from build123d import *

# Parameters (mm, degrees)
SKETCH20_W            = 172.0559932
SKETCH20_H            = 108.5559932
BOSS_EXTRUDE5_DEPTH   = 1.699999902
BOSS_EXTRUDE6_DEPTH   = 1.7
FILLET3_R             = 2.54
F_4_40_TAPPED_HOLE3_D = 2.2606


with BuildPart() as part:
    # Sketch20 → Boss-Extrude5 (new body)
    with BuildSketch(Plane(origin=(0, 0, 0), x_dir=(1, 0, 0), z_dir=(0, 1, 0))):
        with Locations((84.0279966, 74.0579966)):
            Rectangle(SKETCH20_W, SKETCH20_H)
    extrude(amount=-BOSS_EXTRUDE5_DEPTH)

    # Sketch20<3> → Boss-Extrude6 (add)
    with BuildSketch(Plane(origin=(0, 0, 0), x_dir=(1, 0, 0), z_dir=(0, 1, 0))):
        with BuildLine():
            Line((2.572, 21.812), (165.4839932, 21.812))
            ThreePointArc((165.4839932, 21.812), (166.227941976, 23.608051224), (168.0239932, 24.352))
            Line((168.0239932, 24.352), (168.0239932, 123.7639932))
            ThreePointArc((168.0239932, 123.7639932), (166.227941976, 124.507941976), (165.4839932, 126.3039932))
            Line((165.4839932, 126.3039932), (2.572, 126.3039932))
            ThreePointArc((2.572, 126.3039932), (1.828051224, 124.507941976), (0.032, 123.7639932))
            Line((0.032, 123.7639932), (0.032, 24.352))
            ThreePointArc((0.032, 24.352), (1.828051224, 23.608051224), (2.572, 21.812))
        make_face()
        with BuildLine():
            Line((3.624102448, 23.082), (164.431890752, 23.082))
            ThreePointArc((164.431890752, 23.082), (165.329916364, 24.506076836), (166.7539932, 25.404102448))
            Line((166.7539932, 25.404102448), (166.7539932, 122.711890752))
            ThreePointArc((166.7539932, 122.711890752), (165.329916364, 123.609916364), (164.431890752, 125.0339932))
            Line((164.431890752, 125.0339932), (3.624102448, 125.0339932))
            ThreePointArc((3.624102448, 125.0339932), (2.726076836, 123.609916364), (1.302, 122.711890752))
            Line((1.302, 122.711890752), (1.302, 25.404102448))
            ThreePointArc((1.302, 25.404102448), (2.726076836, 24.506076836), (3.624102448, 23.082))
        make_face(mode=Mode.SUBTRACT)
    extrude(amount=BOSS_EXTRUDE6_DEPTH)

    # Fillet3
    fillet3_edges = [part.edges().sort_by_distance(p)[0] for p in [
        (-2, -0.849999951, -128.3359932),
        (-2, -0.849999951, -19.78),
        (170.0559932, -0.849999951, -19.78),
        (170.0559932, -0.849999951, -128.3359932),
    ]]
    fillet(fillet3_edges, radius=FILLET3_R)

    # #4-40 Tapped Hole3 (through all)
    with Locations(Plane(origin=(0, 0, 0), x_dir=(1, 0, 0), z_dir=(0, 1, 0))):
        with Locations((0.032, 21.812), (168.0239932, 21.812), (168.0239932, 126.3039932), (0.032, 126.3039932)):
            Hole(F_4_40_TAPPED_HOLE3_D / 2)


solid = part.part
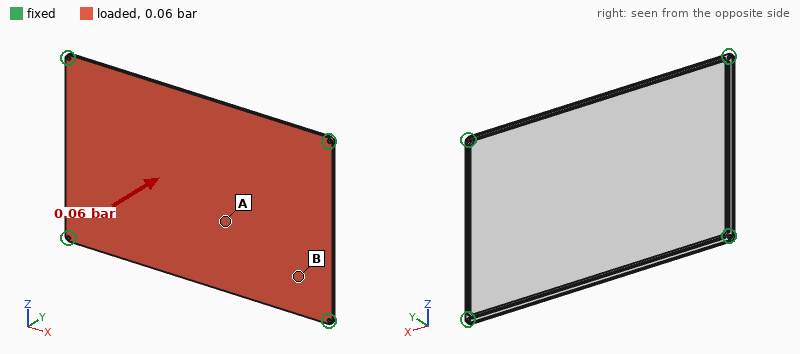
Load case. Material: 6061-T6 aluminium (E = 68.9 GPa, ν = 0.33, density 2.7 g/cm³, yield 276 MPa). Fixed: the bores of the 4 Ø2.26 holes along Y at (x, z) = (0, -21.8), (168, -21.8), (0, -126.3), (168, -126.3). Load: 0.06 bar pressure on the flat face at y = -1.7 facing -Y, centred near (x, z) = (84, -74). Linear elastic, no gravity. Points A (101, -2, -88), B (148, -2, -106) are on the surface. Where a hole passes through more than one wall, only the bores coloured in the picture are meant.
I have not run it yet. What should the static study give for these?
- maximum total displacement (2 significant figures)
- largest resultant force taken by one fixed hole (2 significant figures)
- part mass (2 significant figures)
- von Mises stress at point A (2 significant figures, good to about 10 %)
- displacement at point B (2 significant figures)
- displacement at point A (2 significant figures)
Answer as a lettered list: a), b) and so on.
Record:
a) 0.72 mm
b) 34 N
c) 89 g
d) 15 MPa
e) 0.24 mm
f) 0.68 mm
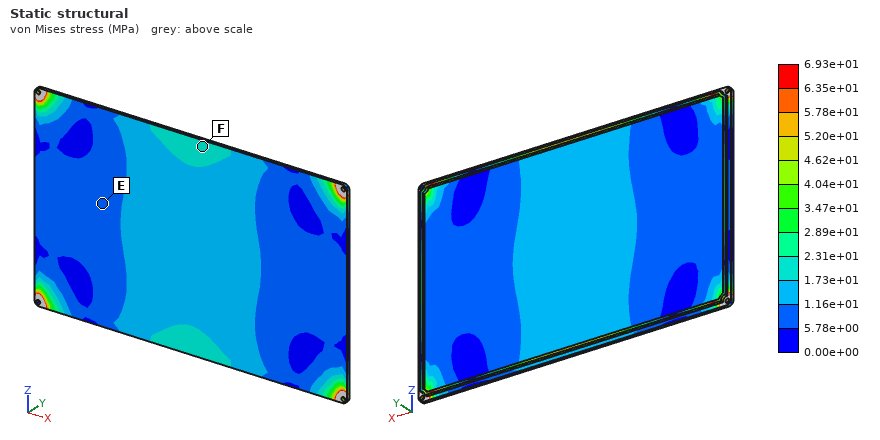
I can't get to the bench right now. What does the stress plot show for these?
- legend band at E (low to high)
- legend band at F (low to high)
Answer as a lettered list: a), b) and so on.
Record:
a) 5.78e+00 to 1.16e+01 MPa
b) 1.73e+01 to 2.31e+01 MPa
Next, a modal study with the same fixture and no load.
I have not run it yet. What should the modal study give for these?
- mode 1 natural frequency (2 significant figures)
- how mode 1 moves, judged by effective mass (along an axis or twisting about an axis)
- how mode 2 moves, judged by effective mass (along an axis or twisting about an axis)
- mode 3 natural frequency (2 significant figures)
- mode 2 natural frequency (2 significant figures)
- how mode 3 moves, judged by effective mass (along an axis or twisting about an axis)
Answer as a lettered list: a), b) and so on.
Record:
a) 240 Hz
b) along Y
c) twisting about X
d) 640 Hz
e) 450 Hz
f) twisting about Z
